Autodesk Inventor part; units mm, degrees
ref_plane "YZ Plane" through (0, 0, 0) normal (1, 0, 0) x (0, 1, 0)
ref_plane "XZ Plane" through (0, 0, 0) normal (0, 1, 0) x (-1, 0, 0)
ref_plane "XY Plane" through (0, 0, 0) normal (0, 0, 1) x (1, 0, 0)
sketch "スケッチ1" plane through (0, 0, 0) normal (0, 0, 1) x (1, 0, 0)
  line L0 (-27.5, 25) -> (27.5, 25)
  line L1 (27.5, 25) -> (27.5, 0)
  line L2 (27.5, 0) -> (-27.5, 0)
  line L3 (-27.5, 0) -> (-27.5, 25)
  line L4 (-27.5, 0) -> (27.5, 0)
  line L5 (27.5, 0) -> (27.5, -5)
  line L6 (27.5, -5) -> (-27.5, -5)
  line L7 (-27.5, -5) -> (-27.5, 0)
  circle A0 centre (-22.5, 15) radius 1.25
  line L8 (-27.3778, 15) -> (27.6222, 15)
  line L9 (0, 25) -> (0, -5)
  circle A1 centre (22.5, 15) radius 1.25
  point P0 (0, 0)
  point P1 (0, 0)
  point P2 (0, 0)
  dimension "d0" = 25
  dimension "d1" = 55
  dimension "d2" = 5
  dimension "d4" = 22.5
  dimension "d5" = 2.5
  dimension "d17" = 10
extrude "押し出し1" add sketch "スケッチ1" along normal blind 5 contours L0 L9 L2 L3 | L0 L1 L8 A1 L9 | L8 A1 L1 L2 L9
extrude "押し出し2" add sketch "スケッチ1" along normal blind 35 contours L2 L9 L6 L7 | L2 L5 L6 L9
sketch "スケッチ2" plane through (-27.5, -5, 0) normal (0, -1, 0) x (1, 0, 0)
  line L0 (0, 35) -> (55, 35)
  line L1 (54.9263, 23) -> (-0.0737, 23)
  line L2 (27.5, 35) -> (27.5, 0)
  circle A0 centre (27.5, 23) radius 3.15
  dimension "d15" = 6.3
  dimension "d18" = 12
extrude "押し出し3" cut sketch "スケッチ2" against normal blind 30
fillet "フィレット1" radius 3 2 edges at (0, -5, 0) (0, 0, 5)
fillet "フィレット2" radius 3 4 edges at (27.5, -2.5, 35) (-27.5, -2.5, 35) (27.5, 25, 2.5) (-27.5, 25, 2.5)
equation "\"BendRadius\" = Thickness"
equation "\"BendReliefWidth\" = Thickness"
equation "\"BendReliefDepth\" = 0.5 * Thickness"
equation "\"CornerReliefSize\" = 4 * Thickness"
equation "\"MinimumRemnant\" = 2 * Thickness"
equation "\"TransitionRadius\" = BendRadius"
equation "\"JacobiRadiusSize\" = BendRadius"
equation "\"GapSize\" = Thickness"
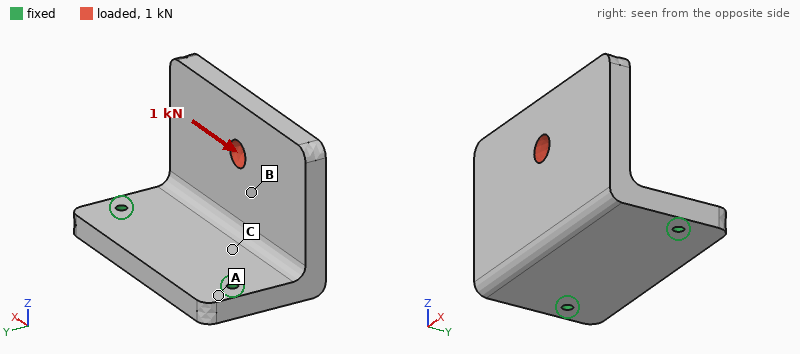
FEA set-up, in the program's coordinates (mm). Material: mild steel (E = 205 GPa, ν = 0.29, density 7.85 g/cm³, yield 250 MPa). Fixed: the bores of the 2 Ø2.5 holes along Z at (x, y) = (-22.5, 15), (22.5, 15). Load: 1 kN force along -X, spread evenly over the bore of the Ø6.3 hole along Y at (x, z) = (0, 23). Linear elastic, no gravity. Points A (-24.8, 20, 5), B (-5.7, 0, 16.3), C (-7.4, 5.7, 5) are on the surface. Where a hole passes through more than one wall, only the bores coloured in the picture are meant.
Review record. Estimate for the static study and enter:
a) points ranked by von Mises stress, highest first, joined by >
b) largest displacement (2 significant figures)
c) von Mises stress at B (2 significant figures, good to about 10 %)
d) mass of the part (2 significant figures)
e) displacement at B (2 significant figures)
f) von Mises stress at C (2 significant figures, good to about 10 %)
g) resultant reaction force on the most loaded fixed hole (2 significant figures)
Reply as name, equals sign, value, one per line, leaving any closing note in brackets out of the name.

points ranked by von Mises stress, highest first, joined by > = C > B > A
largest displacement = 27 µm
von Mises stress at B = 18 MPa
mass of the part = 130 g
displacement at B = 10 µm
von Mises stress at C = 29 MPa
resultant reaction force on the most loaded fixed hole = 780 N
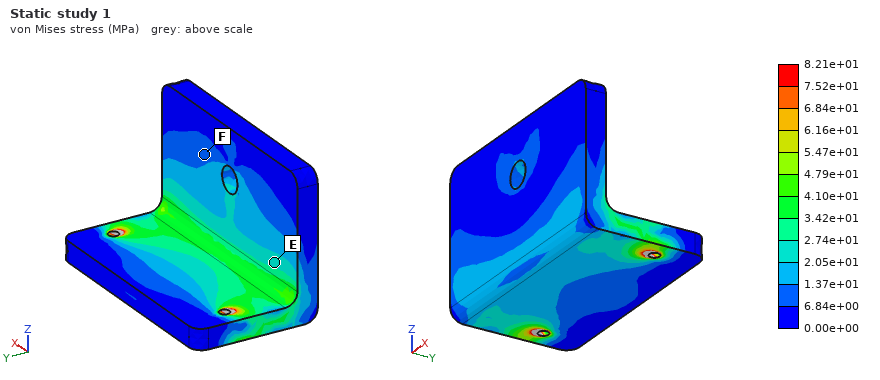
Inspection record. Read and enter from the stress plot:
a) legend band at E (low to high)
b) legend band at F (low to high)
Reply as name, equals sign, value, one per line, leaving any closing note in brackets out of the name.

legend band at E = 2.05e+01 to 2.74e+01 MPa
legend band at F = 6.84e+00 to 1.37e+01 MPa
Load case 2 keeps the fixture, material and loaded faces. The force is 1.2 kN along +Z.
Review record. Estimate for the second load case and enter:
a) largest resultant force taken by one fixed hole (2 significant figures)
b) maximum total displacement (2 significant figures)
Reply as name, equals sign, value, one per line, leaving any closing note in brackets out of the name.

largest resultant force taken by one fixed hole = 600 N
maximum total displacement = 92 µm
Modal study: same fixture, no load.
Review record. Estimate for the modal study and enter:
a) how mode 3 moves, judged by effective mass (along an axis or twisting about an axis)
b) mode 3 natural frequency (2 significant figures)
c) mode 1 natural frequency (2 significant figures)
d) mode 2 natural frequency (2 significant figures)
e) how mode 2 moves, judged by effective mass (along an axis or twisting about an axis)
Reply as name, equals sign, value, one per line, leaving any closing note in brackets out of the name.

how mode 3 moves, judged by effective mass = along Z
mode 3 natural frequency = 5700 Hz
mode 1 natural frequency = 1900 Hz
mode 2 natural frequency = 4100 Hz
how mode 2 moves, judged by effective mass = along X
